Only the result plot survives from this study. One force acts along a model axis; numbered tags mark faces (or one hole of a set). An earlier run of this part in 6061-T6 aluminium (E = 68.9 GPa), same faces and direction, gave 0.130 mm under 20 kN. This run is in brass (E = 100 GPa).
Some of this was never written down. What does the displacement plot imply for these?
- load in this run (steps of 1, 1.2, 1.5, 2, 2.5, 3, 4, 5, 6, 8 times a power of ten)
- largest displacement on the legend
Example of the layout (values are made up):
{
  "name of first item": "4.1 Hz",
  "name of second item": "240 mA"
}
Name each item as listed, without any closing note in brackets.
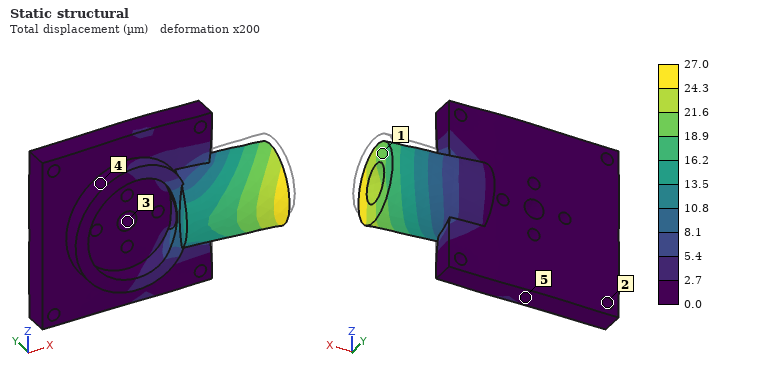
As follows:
{
  "load in this run": "6 kN",
  "largest displacement on the legend": "27.0 µm"
}
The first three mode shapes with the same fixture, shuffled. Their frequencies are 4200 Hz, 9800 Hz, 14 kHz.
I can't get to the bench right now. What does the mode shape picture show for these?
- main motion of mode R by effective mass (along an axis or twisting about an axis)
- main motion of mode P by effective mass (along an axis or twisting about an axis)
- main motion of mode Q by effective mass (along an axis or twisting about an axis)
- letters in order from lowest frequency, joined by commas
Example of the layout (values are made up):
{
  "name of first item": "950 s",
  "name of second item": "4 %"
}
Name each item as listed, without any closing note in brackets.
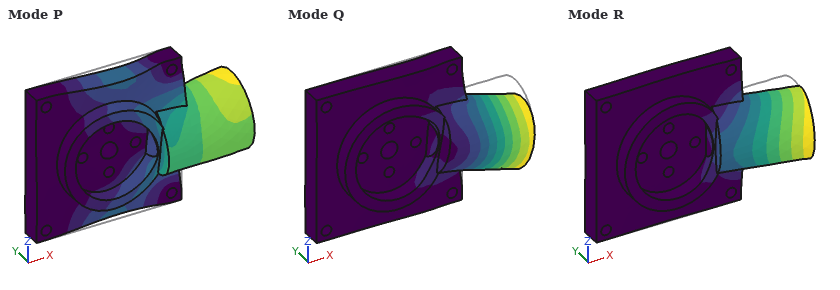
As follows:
{
  "main motion of mode R by effective mass": "along Y",
  "main motion of mode P by effective mass": "twisting about X",
  "main motion of mode Q by effective mass": "along Z",
  "letters in order from lowest frequency, joined by commas": "R, Q, P"
}
